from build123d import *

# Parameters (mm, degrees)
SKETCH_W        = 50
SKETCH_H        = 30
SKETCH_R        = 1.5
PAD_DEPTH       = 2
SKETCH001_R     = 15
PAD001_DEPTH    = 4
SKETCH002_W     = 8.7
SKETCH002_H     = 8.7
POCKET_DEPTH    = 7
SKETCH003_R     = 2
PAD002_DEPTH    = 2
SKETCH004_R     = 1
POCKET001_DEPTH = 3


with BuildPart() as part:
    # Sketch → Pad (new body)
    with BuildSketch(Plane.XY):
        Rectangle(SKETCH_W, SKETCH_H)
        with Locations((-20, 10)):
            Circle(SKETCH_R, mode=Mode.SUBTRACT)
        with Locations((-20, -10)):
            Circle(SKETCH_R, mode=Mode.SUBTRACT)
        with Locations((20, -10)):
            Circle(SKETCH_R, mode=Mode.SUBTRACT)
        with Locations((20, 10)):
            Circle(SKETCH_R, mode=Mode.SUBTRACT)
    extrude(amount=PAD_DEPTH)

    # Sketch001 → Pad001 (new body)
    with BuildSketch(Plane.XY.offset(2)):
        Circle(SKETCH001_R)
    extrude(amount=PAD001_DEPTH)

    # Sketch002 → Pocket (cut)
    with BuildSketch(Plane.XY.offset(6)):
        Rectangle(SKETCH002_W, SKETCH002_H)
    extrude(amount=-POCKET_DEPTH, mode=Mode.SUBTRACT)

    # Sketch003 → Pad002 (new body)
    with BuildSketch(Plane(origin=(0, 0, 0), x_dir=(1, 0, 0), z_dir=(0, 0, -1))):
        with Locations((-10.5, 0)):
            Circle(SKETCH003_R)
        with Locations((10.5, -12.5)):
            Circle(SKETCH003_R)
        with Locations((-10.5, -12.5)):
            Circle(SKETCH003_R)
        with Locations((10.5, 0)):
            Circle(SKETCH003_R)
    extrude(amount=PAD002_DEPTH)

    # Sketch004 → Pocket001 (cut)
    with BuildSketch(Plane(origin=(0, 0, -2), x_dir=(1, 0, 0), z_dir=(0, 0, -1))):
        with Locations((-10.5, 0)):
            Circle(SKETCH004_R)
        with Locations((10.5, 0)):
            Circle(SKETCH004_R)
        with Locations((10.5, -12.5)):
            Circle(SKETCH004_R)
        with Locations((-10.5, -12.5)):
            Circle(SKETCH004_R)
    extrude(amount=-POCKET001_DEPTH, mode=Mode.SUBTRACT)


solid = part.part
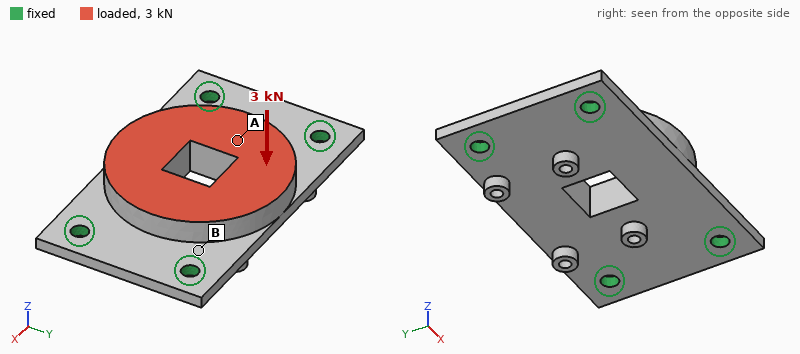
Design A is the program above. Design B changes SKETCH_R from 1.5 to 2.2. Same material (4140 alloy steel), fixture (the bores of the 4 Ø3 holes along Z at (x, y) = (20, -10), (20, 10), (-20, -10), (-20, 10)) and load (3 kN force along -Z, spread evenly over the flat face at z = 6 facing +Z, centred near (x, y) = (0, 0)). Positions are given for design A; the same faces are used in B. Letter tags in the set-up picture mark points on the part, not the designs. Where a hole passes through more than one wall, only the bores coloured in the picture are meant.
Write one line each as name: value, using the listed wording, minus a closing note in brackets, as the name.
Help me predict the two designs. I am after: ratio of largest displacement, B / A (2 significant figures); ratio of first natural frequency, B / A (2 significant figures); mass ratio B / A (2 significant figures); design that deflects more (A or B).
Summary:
ratio of largest displacement, B / A: 0.80
ratio of first natural frequency, B / A: 1.1
mass ratio B / A: 0.99
design that deflects more: A
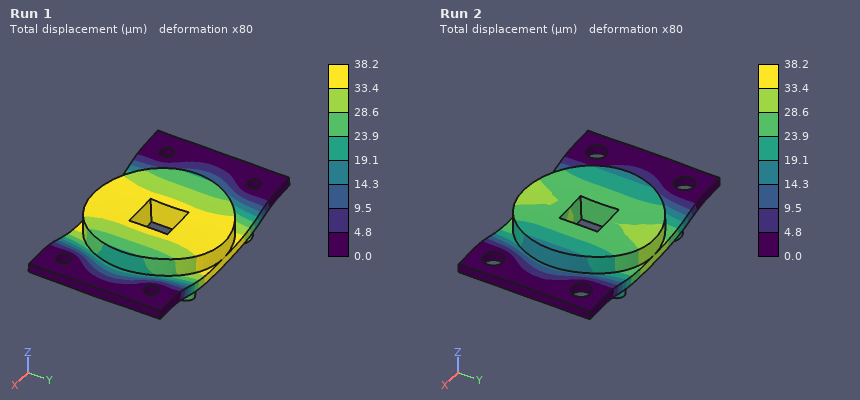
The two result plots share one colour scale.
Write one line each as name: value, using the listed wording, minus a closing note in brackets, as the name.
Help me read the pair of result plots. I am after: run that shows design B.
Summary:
run that shows design B: Run 2
